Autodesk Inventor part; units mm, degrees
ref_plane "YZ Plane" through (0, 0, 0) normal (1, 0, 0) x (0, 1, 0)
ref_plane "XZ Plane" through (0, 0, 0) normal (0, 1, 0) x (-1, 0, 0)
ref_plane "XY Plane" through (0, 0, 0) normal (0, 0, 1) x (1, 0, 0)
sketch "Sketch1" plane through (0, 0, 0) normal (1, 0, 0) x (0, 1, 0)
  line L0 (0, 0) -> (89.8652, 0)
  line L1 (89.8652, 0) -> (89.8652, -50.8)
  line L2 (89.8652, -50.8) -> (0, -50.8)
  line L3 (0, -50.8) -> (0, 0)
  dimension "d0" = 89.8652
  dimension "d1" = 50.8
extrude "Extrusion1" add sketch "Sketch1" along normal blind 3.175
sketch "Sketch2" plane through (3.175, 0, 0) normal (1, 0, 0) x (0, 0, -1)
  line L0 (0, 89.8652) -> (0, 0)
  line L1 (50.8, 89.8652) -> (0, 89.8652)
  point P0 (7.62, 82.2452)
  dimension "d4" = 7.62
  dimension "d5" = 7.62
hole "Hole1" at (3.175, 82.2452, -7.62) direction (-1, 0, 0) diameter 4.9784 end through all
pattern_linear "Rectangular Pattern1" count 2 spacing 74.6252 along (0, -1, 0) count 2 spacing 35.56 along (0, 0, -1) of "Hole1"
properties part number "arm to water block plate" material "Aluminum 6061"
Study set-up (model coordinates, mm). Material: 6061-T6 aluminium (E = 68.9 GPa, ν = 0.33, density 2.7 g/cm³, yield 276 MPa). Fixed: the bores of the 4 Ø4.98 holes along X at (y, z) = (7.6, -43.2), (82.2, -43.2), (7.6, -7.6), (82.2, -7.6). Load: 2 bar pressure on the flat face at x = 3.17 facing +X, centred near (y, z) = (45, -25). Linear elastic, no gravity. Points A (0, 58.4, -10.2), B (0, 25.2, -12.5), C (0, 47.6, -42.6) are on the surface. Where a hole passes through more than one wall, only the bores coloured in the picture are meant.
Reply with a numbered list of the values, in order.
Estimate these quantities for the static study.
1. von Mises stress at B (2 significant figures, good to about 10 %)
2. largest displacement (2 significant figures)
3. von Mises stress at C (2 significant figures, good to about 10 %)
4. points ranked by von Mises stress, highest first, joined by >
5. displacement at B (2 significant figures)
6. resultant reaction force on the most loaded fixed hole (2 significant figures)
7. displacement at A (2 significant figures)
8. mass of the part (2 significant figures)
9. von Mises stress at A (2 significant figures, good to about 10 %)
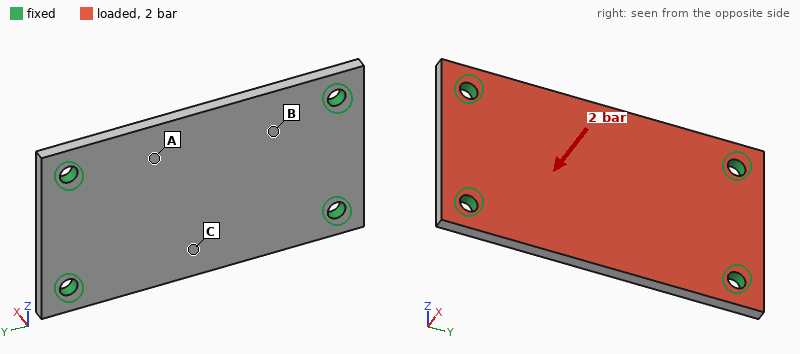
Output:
1. 7.4 MPa
2. 91 µm
3. 26 MPa
4. C > A > B
5. 48 µm
6. 220 N
7. 67 µm
8. 38 g
9. 17 MPa
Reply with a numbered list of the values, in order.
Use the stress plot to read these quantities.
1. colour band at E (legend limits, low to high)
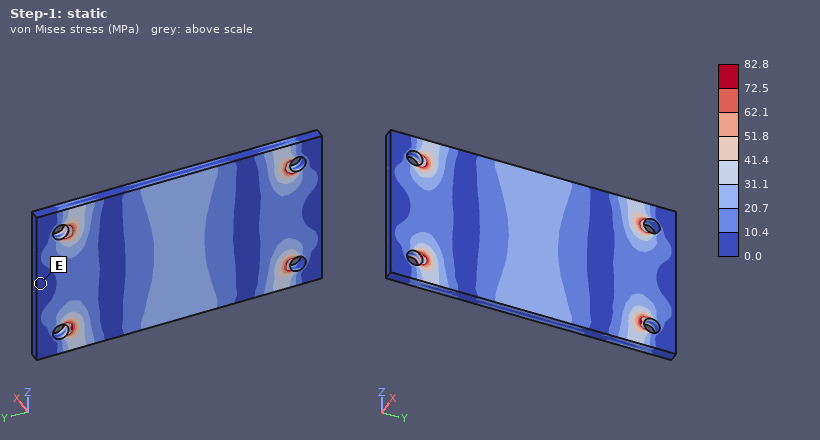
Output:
1. 0.0 to 10.4 MPa
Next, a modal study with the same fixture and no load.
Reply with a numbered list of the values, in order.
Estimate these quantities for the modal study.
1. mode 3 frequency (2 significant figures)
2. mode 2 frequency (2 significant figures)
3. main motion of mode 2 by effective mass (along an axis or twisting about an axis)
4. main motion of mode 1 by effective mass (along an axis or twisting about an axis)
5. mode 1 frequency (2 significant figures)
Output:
1. 7800 Hz
2. 4300 Hz
3. twisting about Y
4. along X
5. 2900 Hz
